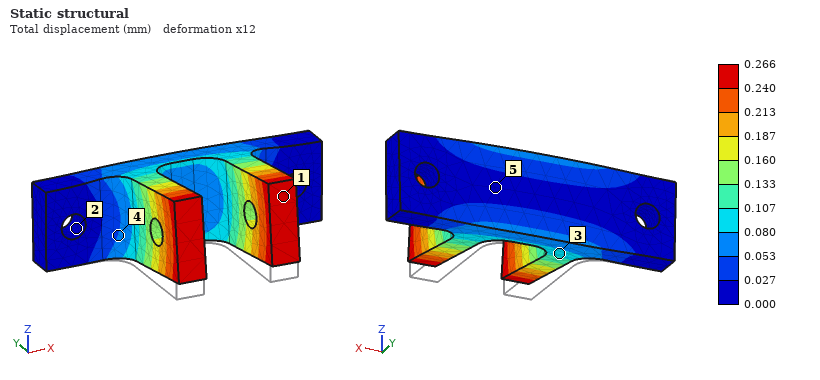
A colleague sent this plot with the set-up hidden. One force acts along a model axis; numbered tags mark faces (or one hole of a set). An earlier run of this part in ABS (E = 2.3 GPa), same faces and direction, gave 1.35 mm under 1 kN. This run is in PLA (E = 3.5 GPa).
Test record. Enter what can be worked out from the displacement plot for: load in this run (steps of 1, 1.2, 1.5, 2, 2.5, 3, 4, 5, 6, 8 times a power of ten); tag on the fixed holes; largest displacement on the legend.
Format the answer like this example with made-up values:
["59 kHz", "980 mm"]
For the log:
["300 N", "2", "0.266 mm"]
